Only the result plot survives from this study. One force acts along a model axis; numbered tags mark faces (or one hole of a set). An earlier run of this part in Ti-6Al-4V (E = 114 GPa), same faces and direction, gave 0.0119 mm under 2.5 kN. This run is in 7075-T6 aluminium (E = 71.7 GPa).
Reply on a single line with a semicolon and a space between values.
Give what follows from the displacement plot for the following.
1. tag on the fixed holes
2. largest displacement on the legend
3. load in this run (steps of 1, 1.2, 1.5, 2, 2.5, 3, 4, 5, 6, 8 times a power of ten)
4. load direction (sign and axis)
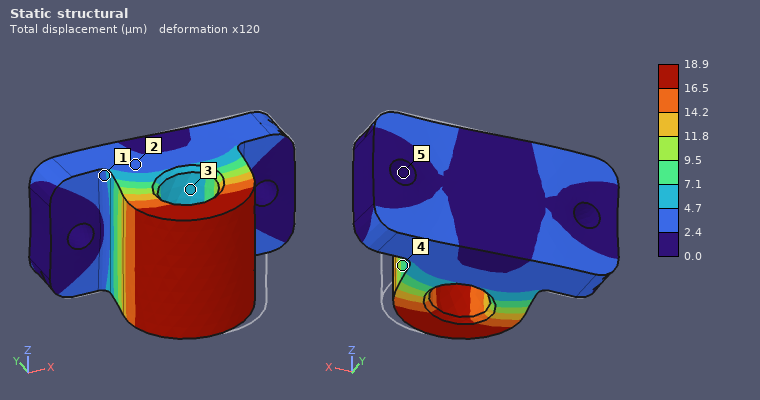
5; 18.9 µm; 2.5 kN; -X
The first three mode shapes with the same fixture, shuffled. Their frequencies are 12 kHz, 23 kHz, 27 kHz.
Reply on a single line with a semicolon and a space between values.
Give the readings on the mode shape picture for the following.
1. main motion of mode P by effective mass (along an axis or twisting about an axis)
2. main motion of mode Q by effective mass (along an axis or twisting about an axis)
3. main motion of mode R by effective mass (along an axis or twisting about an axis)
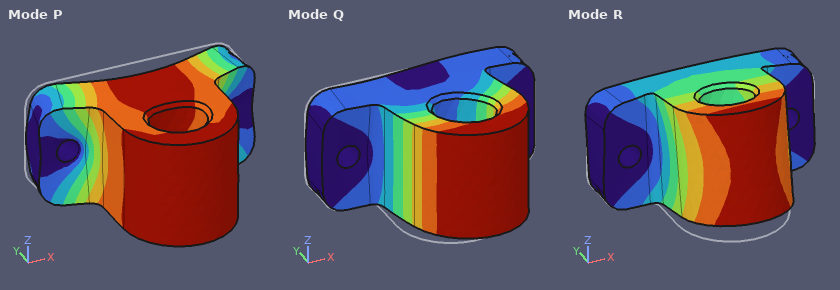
along Y; along X; along Z
